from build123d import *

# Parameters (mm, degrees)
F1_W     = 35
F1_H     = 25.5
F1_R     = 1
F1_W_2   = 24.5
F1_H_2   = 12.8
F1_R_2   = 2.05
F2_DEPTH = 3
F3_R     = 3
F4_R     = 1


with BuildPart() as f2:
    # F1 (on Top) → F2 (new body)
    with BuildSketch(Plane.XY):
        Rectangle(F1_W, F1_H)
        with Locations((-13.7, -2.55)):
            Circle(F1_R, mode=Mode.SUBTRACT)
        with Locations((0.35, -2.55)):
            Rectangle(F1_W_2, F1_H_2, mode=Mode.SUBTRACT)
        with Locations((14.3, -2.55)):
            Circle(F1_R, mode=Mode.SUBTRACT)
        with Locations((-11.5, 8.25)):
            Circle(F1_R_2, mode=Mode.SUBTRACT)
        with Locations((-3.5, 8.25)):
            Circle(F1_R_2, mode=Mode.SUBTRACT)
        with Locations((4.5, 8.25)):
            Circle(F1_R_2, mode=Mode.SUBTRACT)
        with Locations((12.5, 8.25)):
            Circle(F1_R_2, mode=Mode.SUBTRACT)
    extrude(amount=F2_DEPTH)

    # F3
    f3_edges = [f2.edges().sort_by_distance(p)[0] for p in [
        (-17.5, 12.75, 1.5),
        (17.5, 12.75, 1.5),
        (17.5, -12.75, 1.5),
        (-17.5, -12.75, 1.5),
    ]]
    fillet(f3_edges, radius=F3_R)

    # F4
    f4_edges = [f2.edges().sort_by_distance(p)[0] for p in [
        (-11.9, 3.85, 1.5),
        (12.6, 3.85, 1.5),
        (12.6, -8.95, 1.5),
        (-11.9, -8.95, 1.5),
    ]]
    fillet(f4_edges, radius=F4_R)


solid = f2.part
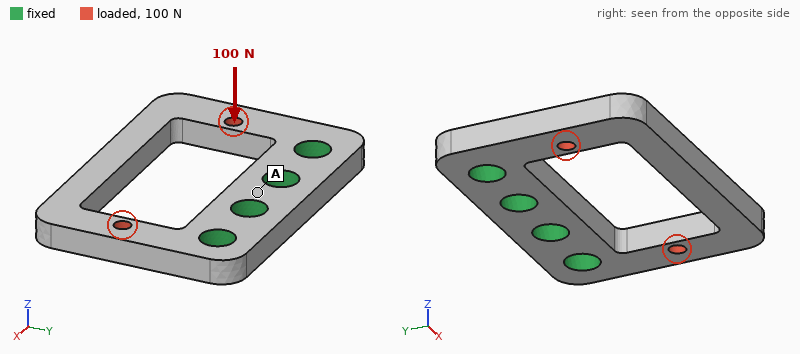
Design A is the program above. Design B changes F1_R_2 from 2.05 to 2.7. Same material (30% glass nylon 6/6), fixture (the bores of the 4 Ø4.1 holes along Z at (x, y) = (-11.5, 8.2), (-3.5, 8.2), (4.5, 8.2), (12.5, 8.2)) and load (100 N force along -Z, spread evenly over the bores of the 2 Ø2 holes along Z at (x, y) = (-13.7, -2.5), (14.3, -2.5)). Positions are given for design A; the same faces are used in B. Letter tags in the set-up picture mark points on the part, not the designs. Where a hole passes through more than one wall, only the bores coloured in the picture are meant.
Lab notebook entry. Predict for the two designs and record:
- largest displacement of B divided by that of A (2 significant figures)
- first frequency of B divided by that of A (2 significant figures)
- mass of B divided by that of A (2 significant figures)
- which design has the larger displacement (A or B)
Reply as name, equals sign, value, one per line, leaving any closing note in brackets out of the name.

largest displacement of B divided by that of A = 0.87
first frequency of B divided by that of A = 1.0
mass of B divided by that of A = 0.92
which design has the larger displacement = A
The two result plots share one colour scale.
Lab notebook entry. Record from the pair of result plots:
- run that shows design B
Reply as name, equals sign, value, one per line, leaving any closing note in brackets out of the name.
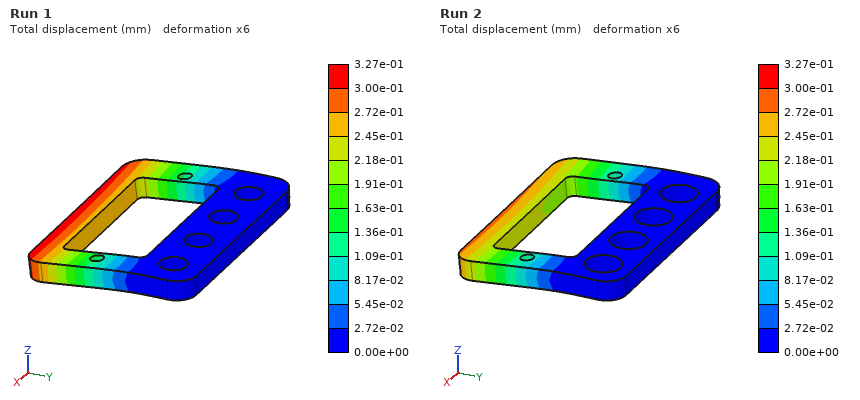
run that shows design B = Run 2
